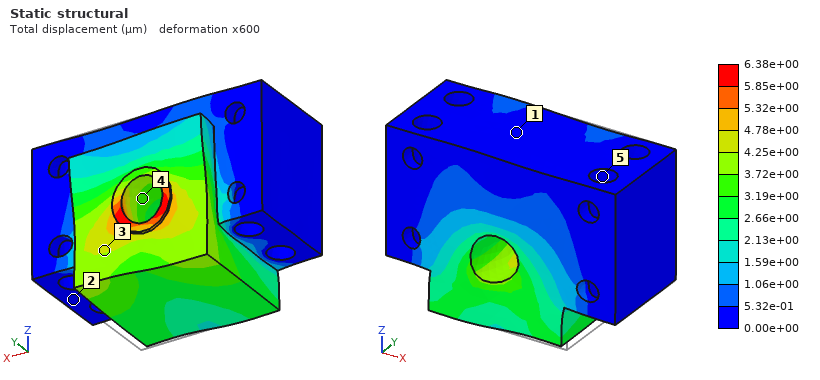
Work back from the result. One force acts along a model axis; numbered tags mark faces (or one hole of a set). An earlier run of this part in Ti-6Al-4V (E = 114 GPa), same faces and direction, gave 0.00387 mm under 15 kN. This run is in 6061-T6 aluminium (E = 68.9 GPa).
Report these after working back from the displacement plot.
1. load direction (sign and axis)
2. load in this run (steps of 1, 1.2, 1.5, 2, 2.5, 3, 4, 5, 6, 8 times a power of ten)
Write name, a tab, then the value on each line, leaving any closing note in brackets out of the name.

load direction	-X
load in this run	15 kN
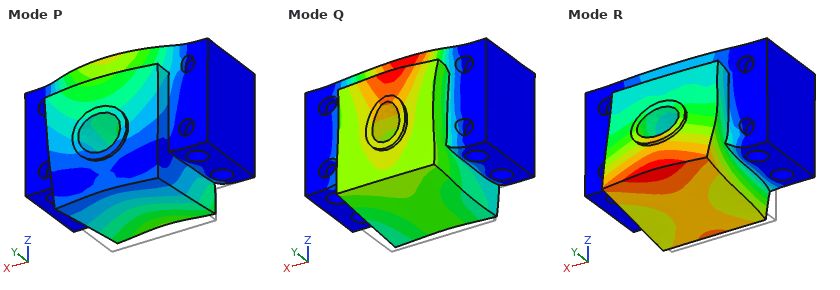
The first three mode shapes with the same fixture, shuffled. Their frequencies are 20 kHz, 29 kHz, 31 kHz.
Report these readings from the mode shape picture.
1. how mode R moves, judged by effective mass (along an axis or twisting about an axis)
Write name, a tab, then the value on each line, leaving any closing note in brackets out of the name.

how mode R moves, judged by effective mass	along Y
